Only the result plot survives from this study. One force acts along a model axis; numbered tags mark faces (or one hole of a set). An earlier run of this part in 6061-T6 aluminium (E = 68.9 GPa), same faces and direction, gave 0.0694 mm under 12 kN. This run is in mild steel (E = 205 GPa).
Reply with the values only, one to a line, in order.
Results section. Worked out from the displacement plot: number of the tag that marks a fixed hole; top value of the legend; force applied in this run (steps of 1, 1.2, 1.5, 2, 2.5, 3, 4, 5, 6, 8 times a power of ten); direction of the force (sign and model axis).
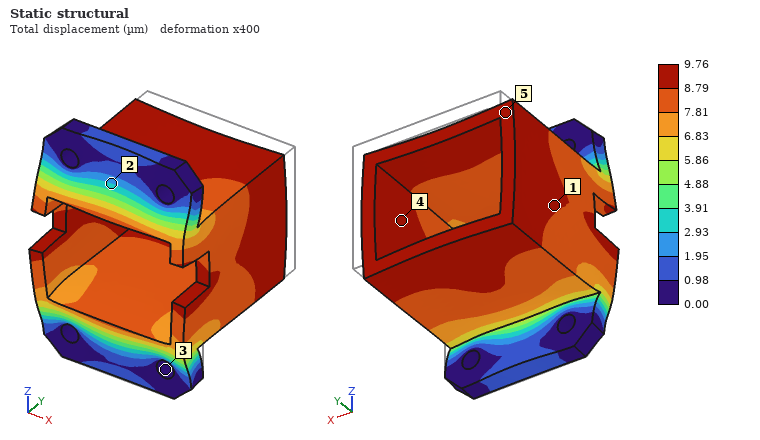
3
9.76 µm
5 kN
-Y
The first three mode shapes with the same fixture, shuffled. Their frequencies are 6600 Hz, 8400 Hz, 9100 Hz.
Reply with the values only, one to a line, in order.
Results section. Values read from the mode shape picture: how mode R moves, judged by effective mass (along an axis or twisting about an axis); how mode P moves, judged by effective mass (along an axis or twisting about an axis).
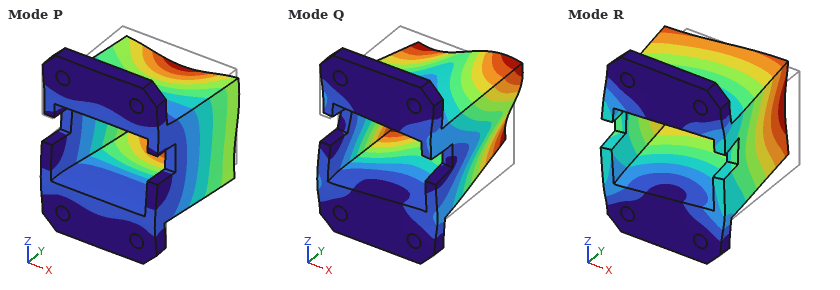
along X
along Z
